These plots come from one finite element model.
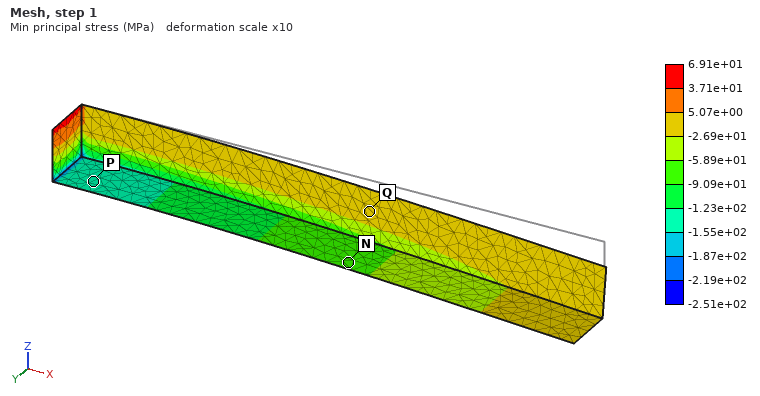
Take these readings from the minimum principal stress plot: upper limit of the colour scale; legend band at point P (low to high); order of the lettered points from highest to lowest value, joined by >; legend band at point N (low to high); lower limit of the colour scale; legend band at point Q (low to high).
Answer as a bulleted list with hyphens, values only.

- 6.91e+01 MPa
- -1.55e+02 to -1.23e+02 MPa
- Q > N > P
- -9.09e+01 to -5.89e+01 MPa
- -2.51e+02 MPa
- -2.69e+01 to 5.07e+00 MPa
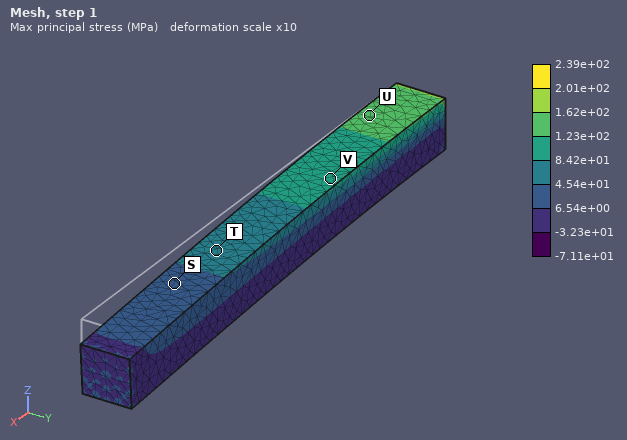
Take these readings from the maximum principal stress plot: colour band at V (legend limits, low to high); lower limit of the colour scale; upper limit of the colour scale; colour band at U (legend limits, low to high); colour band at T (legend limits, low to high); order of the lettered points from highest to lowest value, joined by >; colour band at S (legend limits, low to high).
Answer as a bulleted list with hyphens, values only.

- 8.42e+01 to 1.23e+02 MPa
- -7.11e+01 MPa
- 2.39e+02 MPa
- 1.23e+02 to 1.62e+02 MPa
- 4.54e+01 to 8.42e+01 MPa
- U > V > T > S
- 6.54e+00 to 4.54e+01 MPa
